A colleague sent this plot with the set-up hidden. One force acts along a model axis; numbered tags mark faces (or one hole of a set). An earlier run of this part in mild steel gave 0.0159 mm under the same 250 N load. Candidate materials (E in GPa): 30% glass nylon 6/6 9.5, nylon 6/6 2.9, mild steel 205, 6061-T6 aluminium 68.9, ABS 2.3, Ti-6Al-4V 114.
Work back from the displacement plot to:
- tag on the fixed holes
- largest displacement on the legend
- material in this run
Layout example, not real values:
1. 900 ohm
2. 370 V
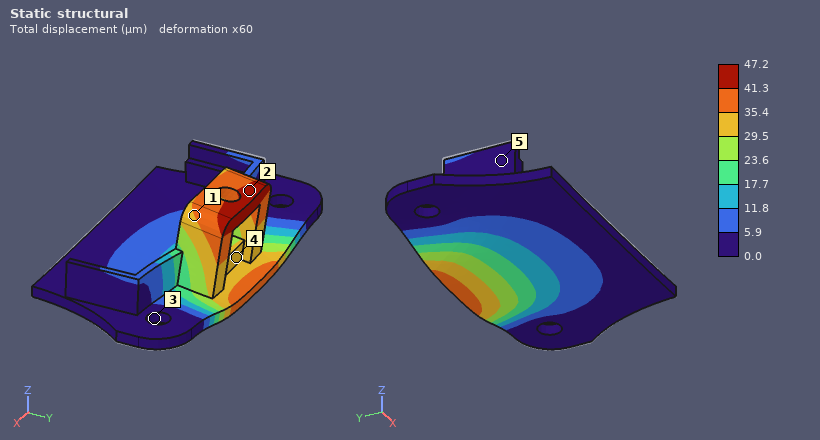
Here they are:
1. 3
2. 47.2 µm
3. 6061-T6 aluminium
